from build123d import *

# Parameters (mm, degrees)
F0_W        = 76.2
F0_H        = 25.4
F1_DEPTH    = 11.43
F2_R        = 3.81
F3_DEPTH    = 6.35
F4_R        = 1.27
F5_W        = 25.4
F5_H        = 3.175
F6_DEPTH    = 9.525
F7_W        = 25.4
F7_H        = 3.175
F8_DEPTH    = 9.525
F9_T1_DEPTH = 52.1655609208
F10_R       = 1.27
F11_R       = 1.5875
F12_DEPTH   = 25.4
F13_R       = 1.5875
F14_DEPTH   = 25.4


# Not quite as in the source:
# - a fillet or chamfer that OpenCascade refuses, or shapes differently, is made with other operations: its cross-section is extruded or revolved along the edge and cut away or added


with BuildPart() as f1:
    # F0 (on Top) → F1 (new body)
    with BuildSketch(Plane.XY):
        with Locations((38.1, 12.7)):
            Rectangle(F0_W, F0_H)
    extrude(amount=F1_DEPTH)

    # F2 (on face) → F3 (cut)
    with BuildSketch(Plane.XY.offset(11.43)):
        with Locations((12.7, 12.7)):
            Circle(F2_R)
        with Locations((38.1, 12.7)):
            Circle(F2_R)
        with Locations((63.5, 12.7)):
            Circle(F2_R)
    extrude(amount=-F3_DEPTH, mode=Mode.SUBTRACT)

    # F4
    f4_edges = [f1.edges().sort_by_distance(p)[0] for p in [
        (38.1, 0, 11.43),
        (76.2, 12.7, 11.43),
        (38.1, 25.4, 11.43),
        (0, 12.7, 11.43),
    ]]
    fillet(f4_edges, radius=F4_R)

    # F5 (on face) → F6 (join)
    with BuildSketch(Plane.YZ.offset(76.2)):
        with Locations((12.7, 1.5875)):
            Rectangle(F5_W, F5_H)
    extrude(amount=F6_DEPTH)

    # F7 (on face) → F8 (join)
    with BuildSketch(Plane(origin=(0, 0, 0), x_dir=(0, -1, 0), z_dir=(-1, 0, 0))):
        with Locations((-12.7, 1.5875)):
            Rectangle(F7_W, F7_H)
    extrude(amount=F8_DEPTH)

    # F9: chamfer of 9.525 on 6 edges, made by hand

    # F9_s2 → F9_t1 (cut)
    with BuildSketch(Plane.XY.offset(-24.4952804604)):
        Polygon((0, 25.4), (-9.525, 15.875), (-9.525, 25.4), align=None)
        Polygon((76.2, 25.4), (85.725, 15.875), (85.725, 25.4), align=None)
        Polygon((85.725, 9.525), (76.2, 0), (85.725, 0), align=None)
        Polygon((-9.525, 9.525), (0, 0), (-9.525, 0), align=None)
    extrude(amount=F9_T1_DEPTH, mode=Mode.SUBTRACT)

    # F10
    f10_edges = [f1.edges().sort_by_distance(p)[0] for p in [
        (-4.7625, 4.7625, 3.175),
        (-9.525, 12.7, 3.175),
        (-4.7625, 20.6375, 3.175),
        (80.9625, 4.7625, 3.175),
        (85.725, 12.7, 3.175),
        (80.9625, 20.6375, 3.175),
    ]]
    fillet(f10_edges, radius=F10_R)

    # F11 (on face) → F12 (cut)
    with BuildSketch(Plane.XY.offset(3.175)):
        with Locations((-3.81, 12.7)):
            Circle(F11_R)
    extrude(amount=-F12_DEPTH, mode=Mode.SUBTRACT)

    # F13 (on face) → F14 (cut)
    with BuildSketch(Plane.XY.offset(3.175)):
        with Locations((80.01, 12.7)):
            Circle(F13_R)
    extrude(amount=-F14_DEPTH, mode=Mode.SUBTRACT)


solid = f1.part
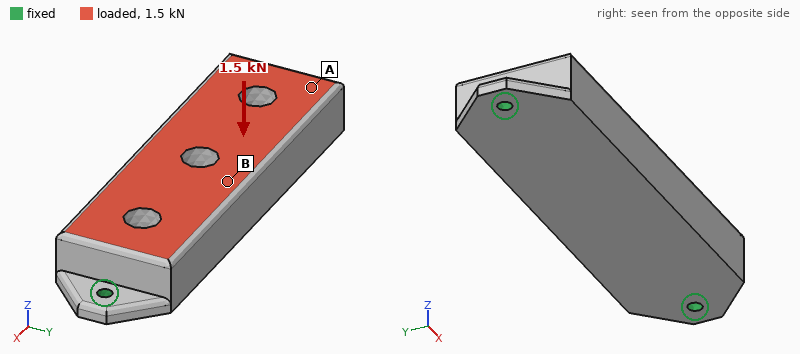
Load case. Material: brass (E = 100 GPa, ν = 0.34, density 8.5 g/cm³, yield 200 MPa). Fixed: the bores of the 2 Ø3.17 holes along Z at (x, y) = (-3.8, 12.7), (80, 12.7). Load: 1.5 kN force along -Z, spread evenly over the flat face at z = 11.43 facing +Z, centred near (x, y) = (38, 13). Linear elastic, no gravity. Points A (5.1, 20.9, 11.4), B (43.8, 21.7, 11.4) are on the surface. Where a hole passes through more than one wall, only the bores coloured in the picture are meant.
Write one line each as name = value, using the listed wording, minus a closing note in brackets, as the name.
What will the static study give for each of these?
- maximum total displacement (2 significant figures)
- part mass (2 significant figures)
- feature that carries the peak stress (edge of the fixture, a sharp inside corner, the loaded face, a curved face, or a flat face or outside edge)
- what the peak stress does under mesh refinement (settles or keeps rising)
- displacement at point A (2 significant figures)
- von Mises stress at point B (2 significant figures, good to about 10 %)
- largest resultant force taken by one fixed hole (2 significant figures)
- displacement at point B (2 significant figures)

maximum total displacement = 30 µm
part mass = 190 g
feature that carries the peak stress = edge of the fixture
what the peak stress does under mesh refinement = keeps rising
displacement at point A = 12 µm
von Mises stress at point B = 27 MPa
largest resultant force taken by one fixed hole = 1.3 kN
displacement at point B = 28 µm
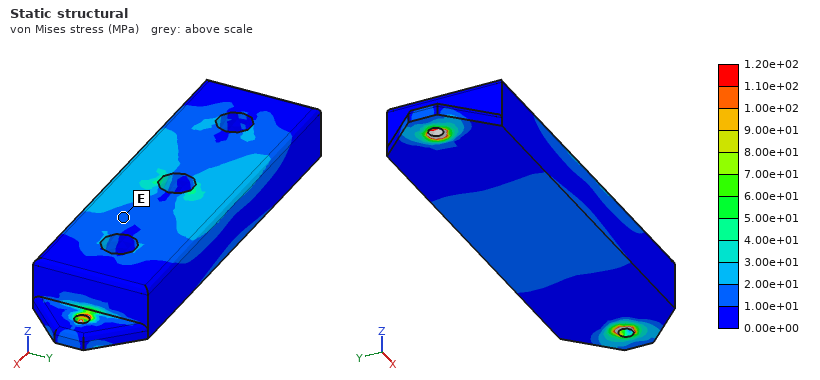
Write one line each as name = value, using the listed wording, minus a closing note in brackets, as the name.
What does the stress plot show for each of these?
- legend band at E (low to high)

legend band at E = 1.00e+01 to 2.00e+01 MPa
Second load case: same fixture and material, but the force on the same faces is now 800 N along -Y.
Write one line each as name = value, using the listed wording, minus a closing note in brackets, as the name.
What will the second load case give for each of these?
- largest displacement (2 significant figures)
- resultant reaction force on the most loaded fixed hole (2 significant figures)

largest displacement = 44 µm
resultant reaction force on the most loaded fixed hole = 400 N
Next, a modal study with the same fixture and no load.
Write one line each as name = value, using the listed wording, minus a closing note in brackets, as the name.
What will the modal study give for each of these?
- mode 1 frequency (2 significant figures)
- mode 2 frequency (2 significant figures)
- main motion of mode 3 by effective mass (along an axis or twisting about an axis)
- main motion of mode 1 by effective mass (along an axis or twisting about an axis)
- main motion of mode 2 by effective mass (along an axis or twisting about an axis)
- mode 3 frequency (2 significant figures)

mode 1 frequency = 2300 Hz
mode 2 frequency = 3000 Hz
main motion of mode 3 by effective mass = along Y
main motion of mode 1 by effective mass = along Y
main motion of mode 2 by effective mass = along Z
mode 3 frequency = 5300 Hz
